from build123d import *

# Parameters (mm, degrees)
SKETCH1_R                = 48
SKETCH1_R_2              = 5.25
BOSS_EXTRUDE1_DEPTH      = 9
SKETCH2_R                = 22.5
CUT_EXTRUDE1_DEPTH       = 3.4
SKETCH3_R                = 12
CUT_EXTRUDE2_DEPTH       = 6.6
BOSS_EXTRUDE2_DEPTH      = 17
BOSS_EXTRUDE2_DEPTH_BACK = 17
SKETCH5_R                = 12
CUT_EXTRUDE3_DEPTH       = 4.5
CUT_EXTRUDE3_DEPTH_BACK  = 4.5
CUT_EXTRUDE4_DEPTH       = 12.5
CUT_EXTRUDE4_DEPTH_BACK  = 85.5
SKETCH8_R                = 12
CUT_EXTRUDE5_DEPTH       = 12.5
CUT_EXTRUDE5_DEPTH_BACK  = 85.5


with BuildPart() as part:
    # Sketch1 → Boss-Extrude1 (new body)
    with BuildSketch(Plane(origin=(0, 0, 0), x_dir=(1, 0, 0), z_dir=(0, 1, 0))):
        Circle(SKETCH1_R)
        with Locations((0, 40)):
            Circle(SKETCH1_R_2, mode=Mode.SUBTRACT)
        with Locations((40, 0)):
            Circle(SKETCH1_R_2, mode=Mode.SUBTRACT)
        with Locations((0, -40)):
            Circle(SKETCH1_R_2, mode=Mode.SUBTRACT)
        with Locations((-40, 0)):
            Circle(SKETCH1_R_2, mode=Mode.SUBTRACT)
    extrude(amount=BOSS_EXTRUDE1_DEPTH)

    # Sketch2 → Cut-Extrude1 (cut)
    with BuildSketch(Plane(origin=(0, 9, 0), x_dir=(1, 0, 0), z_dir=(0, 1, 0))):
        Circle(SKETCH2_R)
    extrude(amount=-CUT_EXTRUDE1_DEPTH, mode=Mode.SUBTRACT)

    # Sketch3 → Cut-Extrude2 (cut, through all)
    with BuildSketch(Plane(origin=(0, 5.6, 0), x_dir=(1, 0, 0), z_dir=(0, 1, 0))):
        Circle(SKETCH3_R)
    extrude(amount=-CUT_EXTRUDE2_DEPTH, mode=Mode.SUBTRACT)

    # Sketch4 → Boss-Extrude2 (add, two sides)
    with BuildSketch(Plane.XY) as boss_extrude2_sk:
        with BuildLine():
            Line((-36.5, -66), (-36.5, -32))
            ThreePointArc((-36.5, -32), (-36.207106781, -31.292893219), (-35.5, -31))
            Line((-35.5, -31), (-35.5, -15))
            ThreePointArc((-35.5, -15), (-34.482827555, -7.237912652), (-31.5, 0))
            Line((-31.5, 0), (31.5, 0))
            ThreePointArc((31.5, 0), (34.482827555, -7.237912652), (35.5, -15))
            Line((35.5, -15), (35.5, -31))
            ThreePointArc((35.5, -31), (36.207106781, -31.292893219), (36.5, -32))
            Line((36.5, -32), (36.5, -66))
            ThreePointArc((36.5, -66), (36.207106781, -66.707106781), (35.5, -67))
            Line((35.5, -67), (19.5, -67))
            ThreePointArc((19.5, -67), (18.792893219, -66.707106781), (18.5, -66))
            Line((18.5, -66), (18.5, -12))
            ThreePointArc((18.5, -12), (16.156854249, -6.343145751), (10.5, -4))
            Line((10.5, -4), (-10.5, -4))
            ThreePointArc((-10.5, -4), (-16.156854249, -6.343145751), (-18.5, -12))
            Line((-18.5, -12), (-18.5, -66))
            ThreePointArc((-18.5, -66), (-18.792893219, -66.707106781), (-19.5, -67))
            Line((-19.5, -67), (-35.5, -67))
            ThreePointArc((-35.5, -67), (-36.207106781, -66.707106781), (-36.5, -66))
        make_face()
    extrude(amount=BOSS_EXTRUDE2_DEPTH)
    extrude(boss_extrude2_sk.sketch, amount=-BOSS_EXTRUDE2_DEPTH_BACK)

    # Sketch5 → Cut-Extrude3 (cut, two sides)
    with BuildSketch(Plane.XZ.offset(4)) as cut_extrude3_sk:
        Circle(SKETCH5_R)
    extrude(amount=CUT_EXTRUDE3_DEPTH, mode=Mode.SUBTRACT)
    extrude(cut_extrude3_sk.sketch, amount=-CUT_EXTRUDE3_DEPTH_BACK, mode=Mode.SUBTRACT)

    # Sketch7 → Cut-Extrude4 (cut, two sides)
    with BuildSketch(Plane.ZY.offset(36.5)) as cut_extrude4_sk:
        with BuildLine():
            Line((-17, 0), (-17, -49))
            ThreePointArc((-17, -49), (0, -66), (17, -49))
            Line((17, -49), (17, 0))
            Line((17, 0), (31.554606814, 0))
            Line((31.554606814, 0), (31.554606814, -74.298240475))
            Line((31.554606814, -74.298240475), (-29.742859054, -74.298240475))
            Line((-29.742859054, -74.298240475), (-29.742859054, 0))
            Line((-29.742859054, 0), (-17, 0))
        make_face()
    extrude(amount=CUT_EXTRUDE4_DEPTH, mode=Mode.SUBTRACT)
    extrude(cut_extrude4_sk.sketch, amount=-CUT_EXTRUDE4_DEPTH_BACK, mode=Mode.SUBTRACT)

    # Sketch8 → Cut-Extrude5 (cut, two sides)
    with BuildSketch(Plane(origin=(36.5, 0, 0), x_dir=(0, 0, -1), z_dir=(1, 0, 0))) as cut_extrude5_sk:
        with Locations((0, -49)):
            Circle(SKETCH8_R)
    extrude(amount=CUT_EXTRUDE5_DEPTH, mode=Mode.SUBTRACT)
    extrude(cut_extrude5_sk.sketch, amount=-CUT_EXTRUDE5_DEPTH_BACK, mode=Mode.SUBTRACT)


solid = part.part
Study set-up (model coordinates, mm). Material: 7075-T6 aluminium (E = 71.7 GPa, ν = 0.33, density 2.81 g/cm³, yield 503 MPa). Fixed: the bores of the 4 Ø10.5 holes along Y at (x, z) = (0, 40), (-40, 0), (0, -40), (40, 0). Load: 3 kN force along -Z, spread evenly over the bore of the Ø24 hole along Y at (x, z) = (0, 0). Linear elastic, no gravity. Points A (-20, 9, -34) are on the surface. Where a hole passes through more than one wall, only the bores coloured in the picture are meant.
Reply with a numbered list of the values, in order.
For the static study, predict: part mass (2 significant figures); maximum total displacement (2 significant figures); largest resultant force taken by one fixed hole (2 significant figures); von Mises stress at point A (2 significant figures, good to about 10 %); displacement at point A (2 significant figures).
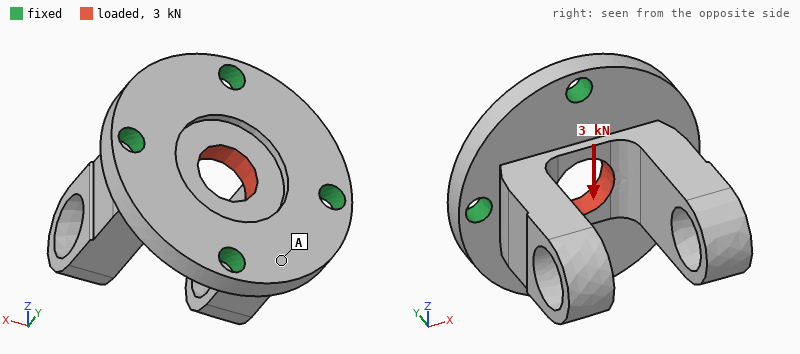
1. 320 g
2. 3.5 µm
3. 940 N
4. 1.3 MPa
5. 0.94 µm
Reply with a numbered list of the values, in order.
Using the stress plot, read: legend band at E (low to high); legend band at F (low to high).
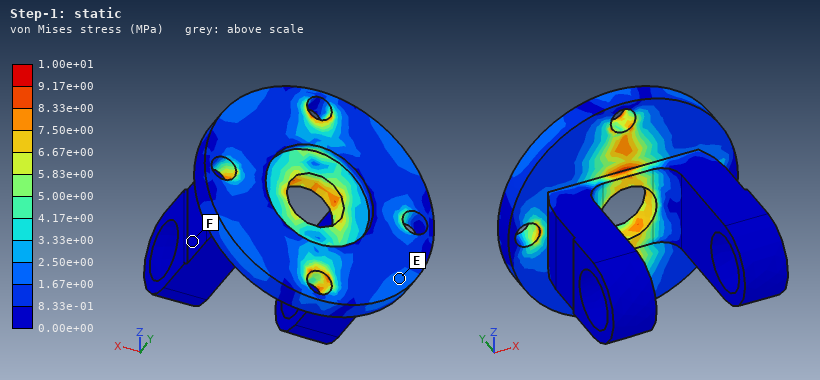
1. 1.67e+00 to 2.50e+00 MPa
2. 0.00e+00 to 8.33e-01 MPa
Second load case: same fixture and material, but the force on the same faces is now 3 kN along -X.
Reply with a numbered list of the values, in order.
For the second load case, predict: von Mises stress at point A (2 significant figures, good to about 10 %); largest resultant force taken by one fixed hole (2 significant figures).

1. 1.0 MPa
2. 1.0 kN
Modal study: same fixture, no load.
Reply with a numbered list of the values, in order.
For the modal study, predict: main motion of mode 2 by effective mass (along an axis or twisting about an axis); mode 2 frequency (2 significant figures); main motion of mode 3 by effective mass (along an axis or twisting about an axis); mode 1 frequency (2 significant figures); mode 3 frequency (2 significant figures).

1. along X
2. 3200 Hz
3. along Z
4. 2800 Hz
5. 3800 Hz
